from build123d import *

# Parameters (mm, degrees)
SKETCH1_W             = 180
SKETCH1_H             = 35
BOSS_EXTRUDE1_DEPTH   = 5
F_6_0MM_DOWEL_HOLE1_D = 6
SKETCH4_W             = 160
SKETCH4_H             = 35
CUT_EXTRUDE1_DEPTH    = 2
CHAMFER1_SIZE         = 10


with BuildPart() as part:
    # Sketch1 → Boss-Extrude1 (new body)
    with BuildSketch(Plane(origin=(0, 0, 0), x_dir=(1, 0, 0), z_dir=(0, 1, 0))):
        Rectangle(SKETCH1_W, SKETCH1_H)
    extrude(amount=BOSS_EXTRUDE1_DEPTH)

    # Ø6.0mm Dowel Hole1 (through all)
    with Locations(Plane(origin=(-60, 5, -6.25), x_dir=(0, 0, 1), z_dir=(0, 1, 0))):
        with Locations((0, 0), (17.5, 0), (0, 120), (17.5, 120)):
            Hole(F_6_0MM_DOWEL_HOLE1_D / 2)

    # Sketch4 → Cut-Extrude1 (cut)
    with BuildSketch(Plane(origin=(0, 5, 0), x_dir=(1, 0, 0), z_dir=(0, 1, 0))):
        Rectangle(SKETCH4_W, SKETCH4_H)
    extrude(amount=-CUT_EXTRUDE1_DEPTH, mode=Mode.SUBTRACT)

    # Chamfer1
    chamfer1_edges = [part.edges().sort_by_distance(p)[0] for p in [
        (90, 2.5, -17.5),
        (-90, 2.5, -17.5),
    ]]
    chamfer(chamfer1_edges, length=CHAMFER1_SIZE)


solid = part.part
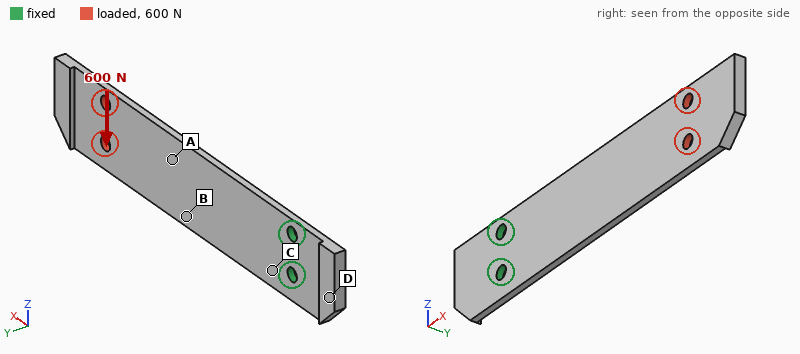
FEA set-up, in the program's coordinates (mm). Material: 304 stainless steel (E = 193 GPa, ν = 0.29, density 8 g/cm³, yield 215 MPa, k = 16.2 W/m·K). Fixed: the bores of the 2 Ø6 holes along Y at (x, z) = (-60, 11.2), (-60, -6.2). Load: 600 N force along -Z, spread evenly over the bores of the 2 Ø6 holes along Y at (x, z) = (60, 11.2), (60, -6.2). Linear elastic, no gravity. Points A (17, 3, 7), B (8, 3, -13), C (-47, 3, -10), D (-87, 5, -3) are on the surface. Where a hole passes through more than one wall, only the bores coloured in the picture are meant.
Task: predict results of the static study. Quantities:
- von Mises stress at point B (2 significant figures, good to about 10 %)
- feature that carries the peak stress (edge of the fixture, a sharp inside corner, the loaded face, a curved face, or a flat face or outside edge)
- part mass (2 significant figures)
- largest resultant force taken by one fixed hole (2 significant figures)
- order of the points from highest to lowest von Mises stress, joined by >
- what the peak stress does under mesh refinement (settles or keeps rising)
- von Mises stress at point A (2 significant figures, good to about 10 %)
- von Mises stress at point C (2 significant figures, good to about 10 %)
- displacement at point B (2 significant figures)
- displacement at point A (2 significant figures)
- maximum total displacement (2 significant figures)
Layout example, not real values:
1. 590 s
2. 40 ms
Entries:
1. 39 MPa
2. edge of the fixture
3. 160 g
4. 3.5 kN
5. C > B > A > D
6. keeps rising
7. 21 MPa
8. 67 MPa
9. 0.081 mm
10. 0.095 mm
11. 0.26 mm
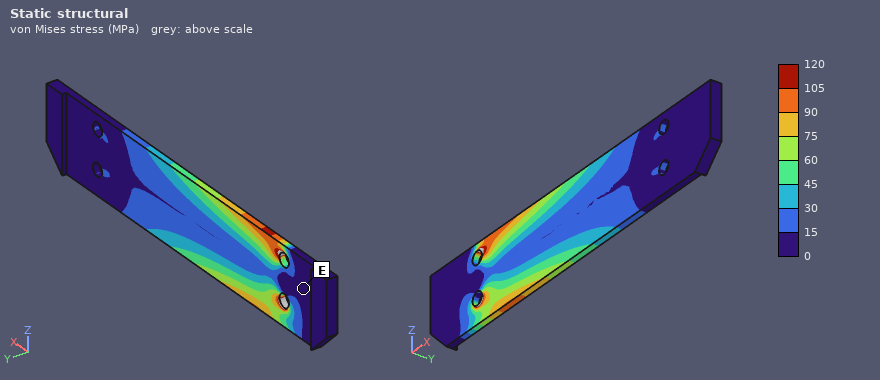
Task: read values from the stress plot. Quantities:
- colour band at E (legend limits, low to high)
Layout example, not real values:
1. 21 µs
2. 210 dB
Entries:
1. 0 to 15 MPa
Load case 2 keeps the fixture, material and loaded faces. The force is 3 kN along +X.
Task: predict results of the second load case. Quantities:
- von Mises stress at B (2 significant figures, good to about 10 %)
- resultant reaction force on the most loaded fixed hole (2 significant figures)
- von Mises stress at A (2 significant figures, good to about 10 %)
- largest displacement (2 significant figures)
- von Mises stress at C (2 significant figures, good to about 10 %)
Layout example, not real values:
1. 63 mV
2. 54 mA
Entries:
1. 19 MPa
2. 1.5 kN
3. 33 MPa
4. 45 µm
5. 23 MPa
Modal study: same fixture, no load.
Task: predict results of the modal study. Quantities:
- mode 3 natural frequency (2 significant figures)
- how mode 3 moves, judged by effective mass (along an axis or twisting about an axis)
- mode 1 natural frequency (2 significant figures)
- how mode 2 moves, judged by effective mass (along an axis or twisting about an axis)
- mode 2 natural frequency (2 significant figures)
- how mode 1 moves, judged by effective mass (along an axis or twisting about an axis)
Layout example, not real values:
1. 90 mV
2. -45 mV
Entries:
1. 900 Hz
2. twisting about X
3. 100 Hz
4. along Y
5. 650 Hz
6. along Y
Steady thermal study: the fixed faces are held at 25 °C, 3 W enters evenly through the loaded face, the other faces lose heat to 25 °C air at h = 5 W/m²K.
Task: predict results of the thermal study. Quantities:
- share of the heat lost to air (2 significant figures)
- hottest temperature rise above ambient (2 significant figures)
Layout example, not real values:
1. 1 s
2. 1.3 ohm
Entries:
1. 77 %
2. 84 K
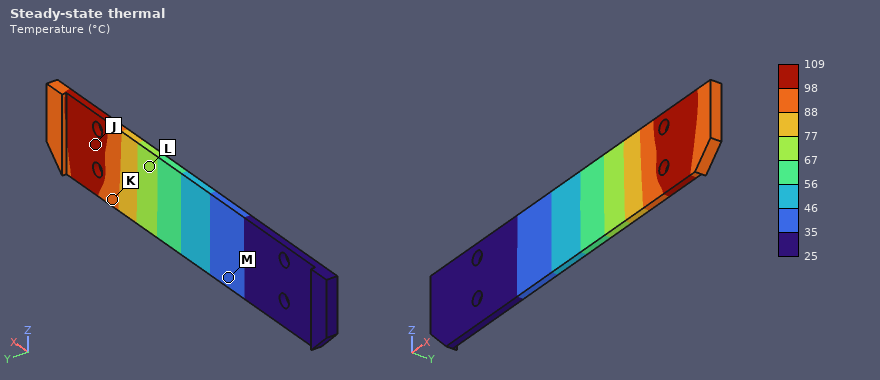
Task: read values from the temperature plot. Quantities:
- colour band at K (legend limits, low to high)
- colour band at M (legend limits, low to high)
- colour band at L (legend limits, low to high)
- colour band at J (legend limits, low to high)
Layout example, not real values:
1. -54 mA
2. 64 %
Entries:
1. 88 to 98 °C
2. 35 to 46 °C
3. 67 to 77 °C
4. 98 to 109 °C
